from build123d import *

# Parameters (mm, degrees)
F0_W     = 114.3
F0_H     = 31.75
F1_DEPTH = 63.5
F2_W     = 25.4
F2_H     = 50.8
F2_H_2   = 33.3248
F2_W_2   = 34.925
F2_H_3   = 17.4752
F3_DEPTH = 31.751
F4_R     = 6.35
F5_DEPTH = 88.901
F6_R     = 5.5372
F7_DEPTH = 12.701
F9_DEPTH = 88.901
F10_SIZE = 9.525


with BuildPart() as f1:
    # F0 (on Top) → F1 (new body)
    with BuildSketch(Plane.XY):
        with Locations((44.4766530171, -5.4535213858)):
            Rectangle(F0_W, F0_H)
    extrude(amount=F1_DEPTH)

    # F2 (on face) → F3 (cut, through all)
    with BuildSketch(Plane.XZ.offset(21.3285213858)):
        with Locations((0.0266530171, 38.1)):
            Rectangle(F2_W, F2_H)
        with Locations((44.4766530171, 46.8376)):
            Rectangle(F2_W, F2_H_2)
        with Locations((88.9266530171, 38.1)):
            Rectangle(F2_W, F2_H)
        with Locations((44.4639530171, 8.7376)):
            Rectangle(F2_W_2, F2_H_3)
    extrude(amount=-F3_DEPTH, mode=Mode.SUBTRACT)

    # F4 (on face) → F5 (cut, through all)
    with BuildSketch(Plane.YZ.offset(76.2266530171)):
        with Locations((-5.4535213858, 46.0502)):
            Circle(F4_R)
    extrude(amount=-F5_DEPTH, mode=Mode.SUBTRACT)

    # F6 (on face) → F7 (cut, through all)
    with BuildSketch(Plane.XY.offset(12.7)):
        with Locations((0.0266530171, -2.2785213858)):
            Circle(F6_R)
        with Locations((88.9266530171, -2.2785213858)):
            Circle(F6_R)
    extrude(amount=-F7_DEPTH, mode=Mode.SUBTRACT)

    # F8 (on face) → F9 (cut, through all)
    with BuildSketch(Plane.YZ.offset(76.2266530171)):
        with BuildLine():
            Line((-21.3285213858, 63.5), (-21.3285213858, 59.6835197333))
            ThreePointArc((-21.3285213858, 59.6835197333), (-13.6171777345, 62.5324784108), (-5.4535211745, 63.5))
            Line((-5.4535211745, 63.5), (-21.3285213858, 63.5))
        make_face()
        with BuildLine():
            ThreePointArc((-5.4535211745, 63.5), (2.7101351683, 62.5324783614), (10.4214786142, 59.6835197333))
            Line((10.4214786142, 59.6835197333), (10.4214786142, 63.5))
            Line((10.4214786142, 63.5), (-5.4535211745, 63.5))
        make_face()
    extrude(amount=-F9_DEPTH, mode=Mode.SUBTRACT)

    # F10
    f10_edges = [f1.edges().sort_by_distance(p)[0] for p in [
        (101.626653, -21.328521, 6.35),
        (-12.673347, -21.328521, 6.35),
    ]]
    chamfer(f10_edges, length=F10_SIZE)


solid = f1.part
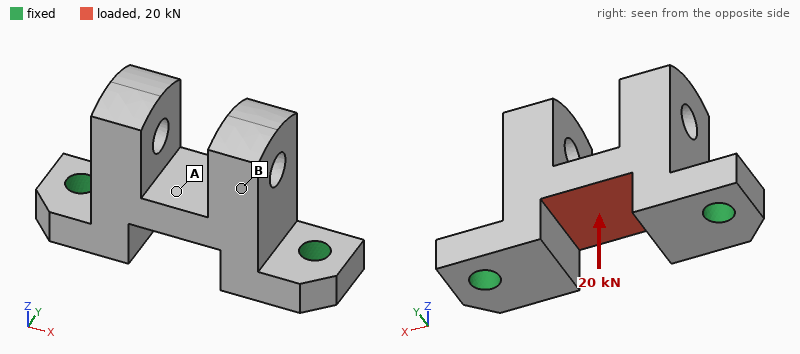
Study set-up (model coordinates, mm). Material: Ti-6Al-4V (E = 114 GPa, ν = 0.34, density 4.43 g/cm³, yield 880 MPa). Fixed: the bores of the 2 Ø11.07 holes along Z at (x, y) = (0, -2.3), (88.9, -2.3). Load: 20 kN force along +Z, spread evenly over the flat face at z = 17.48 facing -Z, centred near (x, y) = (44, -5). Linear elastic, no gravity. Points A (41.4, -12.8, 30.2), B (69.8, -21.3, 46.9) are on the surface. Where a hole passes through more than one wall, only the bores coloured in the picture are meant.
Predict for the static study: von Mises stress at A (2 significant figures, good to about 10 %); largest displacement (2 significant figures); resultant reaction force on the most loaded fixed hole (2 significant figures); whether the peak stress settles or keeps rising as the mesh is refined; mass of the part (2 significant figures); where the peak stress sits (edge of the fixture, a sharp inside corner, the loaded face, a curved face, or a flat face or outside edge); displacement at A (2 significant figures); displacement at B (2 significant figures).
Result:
92 MPa
61 µm
14 kN
keeps rising
410 g
edge of the fixture
48 µm
42 µm
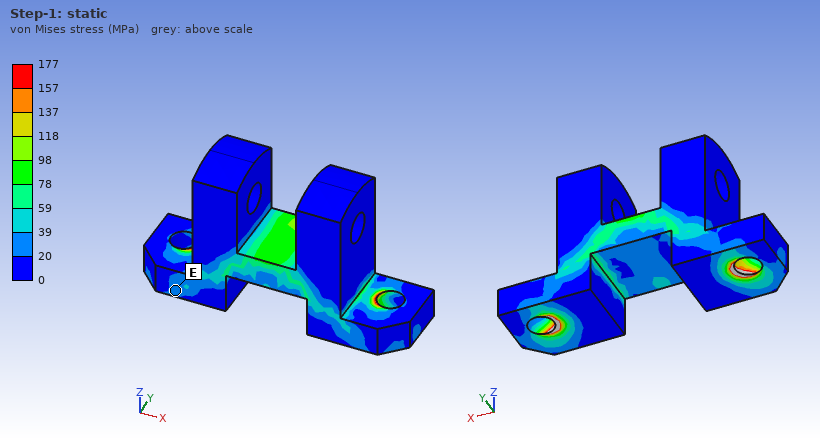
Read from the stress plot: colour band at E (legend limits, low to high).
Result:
20 to 39 MPa
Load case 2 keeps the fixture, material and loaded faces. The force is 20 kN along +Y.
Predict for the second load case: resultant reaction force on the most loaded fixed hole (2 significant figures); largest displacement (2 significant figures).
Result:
10 kN
0.15 mm
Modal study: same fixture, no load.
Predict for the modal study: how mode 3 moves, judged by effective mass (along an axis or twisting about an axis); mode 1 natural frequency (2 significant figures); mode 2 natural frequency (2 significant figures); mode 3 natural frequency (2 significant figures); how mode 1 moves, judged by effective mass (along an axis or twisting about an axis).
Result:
along X
2700 Hz
4600 Hz
5700 Hz
along Y
